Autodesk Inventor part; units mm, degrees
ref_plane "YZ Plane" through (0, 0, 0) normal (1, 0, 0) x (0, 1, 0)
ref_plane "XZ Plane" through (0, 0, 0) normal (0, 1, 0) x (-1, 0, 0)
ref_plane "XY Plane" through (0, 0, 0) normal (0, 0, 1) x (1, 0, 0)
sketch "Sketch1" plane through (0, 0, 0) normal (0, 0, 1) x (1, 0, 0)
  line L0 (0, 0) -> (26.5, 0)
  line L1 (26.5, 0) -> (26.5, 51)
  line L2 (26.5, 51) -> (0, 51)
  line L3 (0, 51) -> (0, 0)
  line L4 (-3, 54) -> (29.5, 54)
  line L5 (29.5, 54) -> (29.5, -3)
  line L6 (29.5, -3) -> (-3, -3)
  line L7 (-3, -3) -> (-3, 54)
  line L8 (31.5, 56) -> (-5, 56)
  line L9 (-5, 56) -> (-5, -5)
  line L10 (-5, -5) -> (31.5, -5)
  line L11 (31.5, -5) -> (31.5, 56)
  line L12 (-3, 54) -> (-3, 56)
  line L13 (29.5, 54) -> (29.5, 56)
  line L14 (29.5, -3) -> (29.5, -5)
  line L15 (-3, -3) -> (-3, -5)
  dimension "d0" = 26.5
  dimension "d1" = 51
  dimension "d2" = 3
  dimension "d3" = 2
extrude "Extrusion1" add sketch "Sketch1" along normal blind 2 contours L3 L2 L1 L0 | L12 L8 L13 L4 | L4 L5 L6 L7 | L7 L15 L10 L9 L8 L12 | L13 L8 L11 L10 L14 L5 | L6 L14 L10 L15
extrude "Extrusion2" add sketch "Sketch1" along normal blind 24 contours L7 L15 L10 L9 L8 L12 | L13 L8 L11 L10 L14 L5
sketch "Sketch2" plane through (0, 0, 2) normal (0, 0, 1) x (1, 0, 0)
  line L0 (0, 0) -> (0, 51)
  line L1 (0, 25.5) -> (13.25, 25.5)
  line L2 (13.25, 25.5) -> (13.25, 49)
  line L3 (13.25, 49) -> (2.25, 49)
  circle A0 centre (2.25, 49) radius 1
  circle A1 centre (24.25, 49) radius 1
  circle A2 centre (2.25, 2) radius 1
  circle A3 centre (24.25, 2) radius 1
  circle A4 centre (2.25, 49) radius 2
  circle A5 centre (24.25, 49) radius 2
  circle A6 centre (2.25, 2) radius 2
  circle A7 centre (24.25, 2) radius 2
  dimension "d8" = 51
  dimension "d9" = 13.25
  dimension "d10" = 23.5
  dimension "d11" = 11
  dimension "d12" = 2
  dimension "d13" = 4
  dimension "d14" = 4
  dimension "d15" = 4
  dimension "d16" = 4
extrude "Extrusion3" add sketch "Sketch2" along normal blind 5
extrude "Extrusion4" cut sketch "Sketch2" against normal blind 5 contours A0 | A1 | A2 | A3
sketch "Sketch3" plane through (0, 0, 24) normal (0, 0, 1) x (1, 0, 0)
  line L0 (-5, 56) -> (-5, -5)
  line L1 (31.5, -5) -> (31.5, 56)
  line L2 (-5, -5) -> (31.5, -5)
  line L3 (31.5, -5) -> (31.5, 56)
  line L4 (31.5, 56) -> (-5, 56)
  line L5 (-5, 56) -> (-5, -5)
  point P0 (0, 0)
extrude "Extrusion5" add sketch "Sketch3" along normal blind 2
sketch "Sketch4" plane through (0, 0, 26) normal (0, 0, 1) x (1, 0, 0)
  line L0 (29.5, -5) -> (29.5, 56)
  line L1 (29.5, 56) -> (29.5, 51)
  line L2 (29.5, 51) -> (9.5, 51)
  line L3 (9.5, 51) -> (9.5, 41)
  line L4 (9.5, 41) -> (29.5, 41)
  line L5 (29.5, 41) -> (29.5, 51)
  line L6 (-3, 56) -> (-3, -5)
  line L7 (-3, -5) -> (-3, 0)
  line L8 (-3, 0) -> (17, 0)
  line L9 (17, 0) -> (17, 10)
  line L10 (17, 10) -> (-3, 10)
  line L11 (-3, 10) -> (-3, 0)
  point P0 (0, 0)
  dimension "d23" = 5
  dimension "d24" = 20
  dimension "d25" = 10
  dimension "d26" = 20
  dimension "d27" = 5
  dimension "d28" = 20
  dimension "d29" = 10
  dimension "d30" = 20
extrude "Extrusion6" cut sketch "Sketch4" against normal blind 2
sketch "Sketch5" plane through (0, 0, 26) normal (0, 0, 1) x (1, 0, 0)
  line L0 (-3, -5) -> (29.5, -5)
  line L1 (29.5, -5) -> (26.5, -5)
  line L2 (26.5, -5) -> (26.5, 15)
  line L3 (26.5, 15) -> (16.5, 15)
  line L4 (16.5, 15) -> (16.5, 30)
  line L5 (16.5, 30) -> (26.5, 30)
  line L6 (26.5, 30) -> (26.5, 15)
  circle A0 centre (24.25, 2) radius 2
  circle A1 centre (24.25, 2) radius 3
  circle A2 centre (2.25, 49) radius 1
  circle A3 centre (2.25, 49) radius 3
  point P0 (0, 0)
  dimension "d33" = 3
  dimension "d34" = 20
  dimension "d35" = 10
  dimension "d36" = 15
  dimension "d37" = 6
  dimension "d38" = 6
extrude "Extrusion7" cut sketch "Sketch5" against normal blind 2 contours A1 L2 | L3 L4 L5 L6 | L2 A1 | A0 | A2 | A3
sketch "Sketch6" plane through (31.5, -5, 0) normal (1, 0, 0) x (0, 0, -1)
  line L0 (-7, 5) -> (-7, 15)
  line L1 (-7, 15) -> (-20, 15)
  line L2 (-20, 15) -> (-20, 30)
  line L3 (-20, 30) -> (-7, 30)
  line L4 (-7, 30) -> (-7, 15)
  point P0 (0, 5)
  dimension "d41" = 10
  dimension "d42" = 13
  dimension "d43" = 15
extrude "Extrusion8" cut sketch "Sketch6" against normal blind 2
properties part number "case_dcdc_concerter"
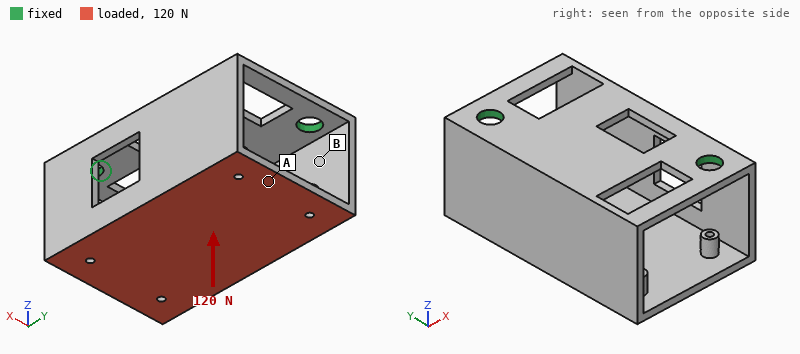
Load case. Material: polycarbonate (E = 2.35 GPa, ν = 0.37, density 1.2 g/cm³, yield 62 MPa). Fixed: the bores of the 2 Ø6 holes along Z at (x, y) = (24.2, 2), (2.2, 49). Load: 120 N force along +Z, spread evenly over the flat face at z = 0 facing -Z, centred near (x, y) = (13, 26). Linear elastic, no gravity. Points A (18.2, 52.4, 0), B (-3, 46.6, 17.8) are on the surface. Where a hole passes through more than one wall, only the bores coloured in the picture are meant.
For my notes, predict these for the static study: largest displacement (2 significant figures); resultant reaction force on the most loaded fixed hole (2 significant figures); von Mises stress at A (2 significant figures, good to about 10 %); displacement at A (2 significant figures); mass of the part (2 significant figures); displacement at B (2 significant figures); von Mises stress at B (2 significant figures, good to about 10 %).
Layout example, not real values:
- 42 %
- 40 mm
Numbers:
- 0.91 mm
- 63 N
- 7.4 MPa
- 0.78 mm
- 15 g
- 0.18 mm
- 4.3 MPa
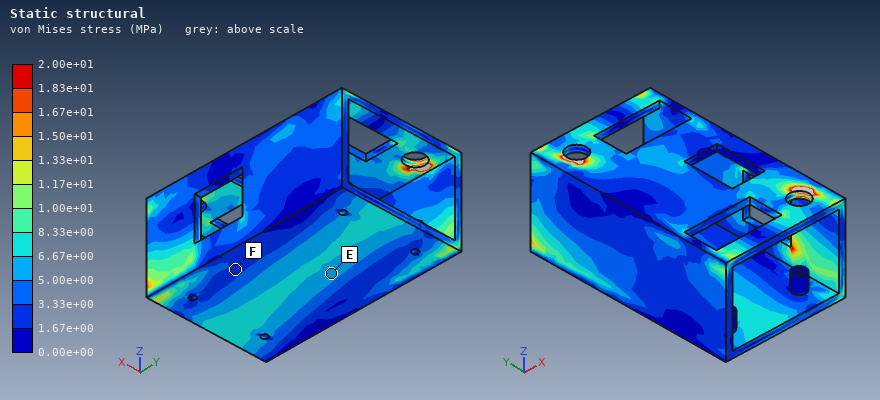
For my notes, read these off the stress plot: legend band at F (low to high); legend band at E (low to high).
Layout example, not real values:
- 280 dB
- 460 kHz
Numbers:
- 1.67e+00 to 3.33e+00 MPa
- 5.00e+00 to 6.67e+00 MPa
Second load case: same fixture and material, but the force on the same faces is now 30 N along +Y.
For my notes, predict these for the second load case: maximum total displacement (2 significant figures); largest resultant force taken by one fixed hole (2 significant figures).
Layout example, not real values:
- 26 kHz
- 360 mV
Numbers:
- 0.84 mm
- 17 N
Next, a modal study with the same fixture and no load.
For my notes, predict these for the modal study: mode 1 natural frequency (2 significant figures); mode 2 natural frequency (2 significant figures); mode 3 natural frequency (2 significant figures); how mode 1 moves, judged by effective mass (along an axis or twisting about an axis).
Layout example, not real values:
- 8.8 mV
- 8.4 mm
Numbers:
- 250 Hz
- 580 Hz
- 600 Hz
- along X
